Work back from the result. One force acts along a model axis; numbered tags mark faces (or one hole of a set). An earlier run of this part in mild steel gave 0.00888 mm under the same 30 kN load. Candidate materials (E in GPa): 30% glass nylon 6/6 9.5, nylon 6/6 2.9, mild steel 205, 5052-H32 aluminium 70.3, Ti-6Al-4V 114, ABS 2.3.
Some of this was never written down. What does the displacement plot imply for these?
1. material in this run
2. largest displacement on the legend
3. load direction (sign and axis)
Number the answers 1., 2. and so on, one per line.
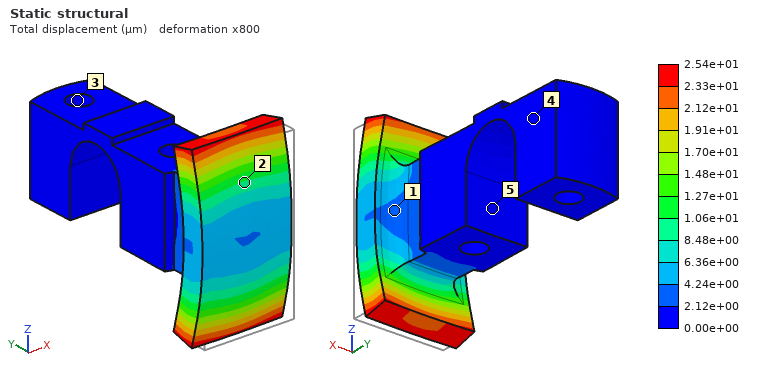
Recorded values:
1. 5052-H32 aluminium
2. 2.54e+01 µm
3. +Y
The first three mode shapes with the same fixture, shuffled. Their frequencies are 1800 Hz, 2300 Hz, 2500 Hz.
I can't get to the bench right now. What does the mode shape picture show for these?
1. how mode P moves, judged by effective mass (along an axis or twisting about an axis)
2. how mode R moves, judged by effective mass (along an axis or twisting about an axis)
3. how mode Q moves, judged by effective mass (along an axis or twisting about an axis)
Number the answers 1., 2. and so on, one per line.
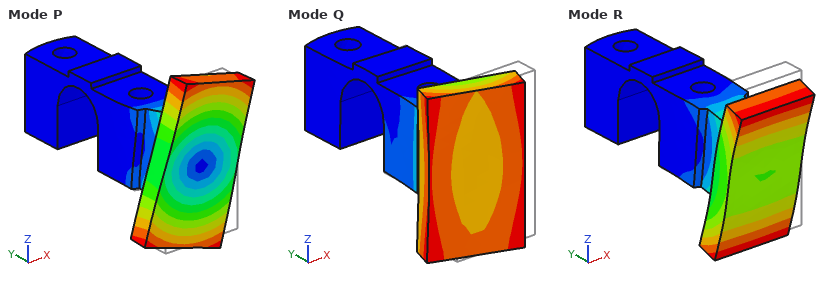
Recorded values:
1. twisting about Y
2. along Z
3. along X
